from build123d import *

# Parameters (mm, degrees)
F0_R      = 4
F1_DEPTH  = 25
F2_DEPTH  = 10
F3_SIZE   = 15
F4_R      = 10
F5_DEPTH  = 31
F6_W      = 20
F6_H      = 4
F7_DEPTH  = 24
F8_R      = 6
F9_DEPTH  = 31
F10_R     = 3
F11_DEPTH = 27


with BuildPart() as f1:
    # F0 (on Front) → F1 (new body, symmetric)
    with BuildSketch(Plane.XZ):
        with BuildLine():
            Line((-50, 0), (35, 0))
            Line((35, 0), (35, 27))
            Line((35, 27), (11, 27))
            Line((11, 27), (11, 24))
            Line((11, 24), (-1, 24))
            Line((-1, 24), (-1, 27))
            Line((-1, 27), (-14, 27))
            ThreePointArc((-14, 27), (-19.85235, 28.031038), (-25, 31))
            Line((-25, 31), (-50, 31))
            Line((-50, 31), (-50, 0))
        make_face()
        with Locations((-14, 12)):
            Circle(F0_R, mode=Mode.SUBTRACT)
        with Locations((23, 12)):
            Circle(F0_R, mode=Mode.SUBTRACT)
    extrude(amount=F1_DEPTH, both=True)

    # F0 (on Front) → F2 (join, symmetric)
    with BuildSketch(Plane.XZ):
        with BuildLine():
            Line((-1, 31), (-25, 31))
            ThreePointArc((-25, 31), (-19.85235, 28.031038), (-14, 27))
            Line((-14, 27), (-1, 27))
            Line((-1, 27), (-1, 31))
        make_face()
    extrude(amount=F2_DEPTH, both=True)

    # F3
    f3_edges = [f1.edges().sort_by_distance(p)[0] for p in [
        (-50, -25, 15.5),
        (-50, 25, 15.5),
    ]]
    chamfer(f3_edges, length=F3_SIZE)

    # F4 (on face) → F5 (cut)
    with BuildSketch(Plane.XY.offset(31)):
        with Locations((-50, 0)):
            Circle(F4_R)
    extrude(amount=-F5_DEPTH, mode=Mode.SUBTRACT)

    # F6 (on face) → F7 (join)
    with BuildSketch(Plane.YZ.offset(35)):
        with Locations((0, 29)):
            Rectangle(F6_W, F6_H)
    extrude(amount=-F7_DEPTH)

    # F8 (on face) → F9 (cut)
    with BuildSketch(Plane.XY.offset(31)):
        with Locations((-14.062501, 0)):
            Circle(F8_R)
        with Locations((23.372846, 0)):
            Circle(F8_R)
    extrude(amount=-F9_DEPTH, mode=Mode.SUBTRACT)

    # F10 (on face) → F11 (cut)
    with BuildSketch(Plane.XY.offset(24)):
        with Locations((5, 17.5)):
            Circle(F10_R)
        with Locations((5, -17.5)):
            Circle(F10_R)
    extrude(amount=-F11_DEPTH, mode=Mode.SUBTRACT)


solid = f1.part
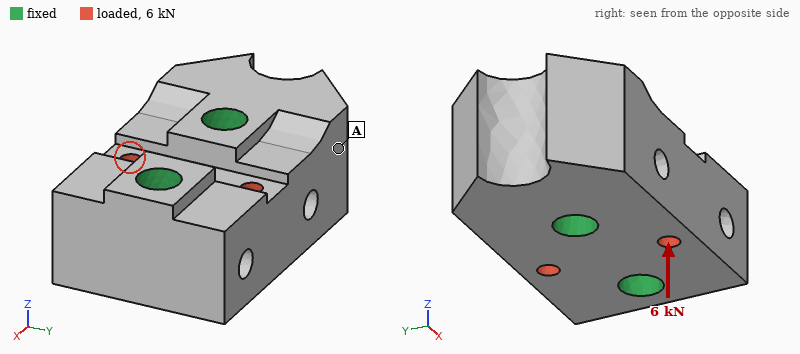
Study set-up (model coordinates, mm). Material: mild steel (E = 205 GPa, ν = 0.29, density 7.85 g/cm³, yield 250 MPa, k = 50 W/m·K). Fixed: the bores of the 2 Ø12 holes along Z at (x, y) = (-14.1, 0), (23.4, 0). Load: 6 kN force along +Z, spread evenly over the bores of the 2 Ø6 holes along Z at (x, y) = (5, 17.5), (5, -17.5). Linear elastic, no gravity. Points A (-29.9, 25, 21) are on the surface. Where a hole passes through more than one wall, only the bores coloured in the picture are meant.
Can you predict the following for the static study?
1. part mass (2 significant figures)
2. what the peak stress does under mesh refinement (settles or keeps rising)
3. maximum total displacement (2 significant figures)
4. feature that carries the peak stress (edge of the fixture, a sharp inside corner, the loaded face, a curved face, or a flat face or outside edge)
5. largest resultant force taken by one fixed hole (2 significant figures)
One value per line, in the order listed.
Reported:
770 g
keeps rising
1.5 µm
a sharp inside corner
3.0 kN
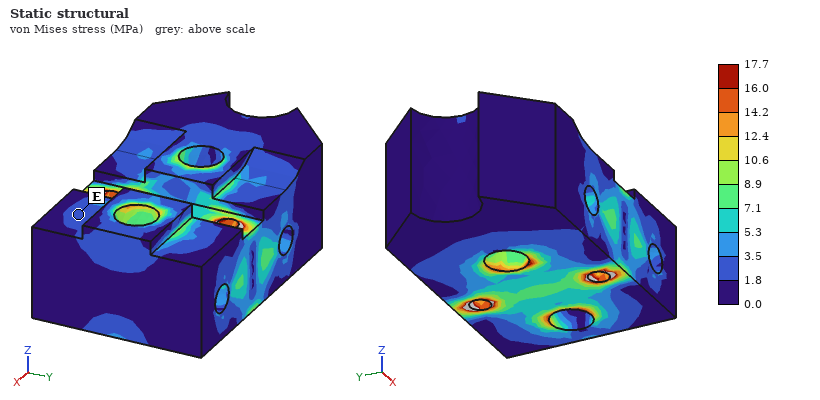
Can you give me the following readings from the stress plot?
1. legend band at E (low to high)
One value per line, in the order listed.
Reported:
1.8 to 3.5 MPa
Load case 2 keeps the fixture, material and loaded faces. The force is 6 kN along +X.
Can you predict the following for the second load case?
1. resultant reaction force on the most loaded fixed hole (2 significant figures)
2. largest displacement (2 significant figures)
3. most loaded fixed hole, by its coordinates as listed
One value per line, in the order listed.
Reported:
3.2 kN
0.73 µm
(-14.1, 0)
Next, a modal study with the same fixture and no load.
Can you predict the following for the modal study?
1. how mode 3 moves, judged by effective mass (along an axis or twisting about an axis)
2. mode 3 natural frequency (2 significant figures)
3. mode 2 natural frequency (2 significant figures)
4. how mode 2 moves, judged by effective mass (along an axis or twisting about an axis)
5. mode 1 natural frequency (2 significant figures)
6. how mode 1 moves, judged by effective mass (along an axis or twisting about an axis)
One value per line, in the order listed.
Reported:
twisting about X
19 kHz
17 kHz
along Z
15 kHz
along Y
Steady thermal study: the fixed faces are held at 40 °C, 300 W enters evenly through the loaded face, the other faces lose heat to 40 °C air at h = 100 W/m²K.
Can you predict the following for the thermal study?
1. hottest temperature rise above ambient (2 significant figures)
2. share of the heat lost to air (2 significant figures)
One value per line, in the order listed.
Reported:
72 K
9.5 %
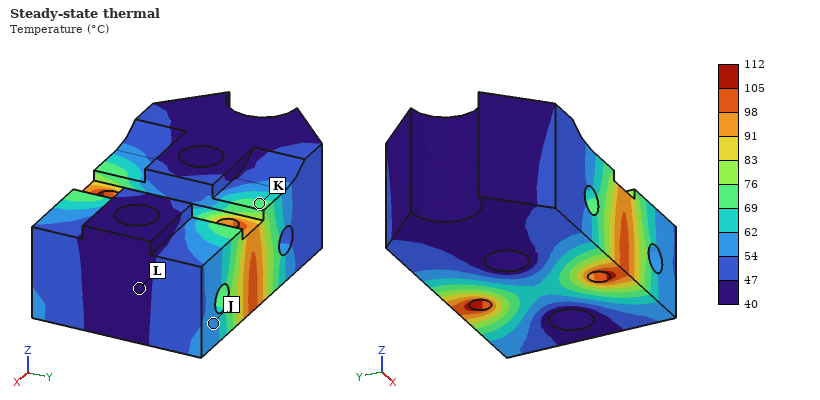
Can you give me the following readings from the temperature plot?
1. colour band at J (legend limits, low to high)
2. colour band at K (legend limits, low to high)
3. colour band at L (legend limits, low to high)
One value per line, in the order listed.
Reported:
54 to 62 °C
69 to 76 °C
40 to 47 °C
